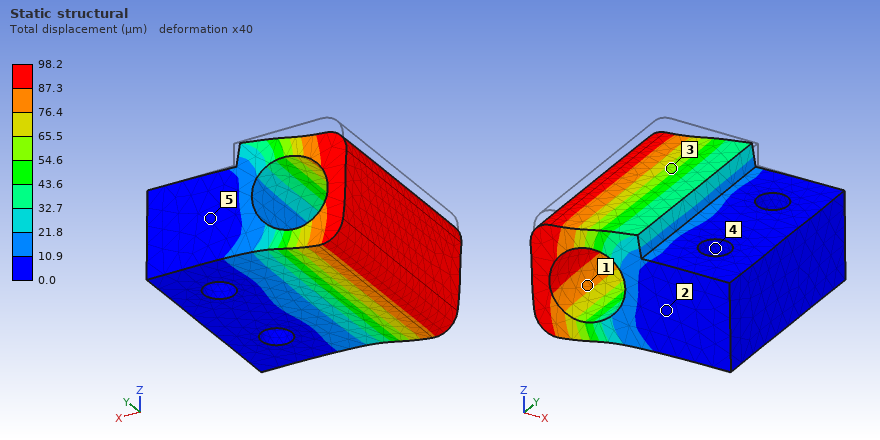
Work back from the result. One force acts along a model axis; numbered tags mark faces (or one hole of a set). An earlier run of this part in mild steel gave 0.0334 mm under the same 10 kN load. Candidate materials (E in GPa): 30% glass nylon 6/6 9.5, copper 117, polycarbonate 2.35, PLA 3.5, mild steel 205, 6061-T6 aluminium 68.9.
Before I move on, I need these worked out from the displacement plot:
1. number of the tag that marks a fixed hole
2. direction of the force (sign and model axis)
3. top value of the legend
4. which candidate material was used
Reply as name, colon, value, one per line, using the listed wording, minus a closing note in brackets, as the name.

number of the tag that marks a fixed hole: 4
direction of the force: -Z
top value of the legend: 98.2 µm
which candidate material was used: 6061-T6 aluminium
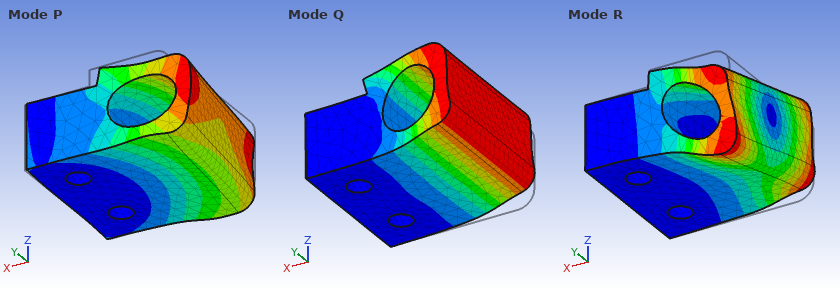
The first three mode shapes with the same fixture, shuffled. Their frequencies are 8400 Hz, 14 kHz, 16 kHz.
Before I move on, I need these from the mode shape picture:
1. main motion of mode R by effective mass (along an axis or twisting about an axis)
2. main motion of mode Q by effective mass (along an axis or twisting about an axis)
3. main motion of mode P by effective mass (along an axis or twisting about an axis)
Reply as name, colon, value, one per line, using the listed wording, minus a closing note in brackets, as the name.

main motion of mode R by effective mass: twisting about X
main motion of mode Q by effective mass: along Z
main motion of mode P by effective mass: along Y
